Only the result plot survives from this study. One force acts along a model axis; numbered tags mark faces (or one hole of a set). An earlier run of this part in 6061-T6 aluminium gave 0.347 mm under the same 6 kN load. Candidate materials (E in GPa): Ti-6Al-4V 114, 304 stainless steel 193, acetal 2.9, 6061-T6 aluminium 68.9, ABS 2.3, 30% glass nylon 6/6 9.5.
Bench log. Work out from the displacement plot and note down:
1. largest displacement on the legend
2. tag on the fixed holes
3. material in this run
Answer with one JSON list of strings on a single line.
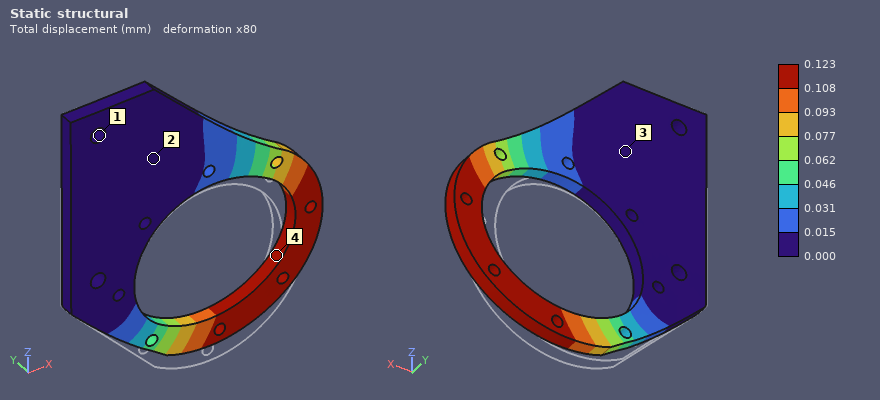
["0.123 mm", "1", "304 stainless steel"]
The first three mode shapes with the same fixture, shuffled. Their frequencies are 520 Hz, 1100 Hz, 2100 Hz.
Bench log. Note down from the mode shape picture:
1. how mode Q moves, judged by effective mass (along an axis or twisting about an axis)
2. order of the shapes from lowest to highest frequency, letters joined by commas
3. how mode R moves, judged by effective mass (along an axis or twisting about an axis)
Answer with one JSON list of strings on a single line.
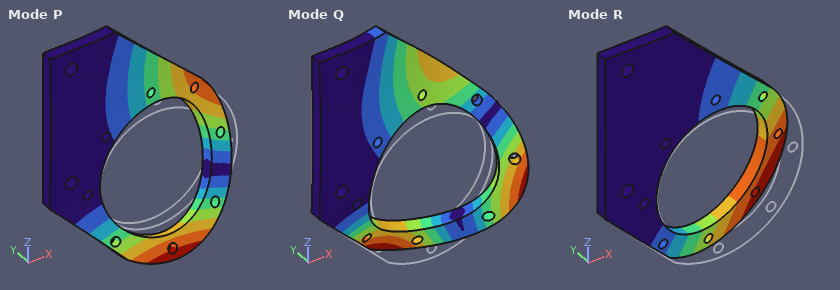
["along Y", "R, P, Q", "along Y"]
